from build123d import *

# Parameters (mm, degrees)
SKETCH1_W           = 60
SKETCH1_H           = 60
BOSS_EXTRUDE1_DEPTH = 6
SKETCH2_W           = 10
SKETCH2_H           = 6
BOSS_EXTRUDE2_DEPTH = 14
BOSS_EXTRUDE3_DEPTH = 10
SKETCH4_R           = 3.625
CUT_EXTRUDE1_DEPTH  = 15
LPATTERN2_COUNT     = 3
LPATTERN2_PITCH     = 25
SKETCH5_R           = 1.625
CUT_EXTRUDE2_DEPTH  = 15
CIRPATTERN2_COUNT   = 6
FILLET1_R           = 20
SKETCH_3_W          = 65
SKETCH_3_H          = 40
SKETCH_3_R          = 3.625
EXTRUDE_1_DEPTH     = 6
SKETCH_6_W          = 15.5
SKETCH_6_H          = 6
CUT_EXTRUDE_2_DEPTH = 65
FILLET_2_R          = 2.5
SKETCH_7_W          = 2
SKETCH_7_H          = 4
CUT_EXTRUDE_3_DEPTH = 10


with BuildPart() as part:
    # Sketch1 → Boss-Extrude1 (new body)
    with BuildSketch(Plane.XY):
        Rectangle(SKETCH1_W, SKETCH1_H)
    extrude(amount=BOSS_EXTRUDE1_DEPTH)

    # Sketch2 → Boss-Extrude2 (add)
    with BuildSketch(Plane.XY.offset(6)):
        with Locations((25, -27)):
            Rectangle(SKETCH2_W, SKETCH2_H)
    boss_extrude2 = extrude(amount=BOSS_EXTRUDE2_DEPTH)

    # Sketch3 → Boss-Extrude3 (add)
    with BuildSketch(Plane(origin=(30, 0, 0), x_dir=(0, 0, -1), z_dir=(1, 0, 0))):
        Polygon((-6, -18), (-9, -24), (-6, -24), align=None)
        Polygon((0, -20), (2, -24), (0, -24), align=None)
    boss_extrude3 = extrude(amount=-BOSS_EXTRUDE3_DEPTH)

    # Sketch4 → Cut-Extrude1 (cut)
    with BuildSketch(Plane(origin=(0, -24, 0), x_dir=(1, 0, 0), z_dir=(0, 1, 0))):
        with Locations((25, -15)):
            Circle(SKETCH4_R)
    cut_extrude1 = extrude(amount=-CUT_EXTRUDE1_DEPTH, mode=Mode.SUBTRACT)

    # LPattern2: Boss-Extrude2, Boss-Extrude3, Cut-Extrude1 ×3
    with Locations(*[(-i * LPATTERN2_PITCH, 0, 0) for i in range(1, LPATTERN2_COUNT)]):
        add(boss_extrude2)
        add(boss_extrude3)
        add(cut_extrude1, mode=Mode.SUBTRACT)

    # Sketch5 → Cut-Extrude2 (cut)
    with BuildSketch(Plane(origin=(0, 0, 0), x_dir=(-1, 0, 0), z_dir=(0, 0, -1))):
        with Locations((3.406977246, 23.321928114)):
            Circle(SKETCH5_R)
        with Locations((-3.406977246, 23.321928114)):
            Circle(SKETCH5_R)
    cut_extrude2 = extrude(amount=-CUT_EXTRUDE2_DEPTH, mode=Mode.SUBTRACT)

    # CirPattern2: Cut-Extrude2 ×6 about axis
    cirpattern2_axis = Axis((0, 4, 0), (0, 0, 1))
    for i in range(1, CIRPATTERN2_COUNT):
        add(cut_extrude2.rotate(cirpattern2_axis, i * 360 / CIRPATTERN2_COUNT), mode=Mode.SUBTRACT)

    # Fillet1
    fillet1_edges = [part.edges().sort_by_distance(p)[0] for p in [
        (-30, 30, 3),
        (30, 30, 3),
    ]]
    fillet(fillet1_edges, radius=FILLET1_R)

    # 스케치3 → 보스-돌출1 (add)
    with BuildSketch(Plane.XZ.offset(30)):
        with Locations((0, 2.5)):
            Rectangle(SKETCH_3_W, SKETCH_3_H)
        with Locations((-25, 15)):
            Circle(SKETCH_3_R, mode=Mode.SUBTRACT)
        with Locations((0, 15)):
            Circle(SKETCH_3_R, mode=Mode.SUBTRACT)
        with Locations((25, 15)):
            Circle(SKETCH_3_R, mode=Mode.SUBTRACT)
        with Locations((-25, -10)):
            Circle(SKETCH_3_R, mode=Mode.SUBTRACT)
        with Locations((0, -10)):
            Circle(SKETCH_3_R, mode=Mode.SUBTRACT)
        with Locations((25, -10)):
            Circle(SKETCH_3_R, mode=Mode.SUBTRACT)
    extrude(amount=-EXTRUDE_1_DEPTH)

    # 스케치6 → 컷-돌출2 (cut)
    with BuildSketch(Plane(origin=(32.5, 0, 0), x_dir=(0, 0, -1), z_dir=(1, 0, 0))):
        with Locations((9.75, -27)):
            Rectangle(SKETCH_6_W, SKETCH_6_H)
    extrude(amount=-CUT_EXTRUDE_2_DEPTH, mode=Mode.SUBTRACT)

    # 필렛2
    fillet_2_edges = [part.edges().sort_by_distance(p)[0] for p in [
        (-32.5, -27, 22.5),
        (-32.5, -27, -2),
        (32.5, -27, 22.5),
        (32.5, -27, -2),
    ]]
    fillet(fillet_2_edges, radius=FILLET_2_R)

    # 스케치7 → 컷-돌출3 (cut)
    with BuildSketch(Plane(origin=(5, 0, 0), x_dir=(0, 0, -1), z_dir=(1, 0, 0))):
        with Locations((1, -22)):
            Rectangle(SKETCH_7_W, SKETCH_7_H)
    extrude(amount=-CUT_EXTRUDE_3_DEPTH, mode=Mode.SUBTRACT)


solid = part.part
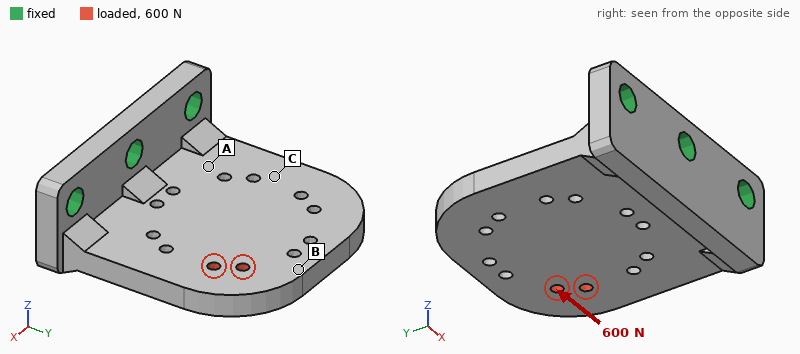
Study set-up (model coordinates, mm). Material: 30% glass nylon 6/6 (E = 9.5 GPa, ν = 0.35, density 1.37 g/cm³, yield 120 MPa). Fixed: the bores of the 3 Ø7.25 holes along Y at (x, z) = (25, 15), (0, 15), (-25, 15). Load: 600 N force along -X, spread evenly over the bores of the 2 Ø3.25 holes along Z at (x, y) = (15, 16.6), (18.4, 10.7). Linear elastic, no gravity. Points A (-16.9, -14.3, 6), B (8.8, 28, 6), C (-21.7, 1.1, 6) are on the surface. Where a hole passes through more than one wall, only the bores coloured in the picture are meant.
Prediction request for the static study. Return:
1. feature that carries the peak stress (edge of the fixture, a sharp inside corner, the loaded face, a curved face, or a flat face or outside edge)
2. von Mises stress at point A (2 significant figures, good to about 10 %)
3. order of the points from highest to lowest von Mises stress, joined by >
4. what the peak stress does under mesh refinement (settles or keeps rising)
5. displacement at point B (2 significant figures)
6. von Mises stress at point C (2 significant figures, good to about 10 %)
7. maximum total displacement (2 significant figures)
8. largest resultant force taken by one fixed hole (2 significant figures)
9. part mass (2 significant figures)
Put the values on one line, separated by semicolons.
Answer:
edge of the fixture; 8.1 MPa; A > C > B; keeps rising; 0.13 mm; 4.6 MPa; 0.15 mm; 510 N; 37 g
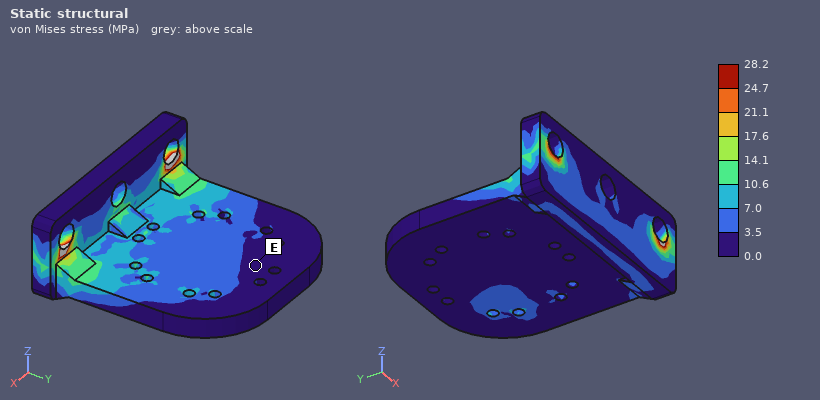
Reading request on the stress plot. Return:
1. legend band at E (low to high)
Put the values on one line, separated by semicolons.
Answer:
0.0 to 3.5 MPa
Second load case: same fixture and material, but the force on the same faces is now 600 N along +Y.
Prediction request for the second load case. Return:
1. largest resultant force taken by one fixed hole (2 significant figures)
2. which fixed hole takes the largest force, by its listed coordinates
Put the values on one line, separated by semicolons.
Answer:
390 N; (25, 15)
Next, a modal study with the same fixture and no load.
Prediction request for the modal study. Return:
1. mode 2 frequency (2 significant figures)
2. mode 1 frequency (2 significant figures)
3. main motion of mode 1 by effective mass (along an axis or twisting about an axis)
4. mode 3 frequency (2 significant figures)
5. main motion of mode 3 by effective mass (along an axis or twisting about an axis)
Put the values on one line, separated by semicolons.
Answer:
2000 Hz; 770 Hz; along Z; 3300 Hz; along X
